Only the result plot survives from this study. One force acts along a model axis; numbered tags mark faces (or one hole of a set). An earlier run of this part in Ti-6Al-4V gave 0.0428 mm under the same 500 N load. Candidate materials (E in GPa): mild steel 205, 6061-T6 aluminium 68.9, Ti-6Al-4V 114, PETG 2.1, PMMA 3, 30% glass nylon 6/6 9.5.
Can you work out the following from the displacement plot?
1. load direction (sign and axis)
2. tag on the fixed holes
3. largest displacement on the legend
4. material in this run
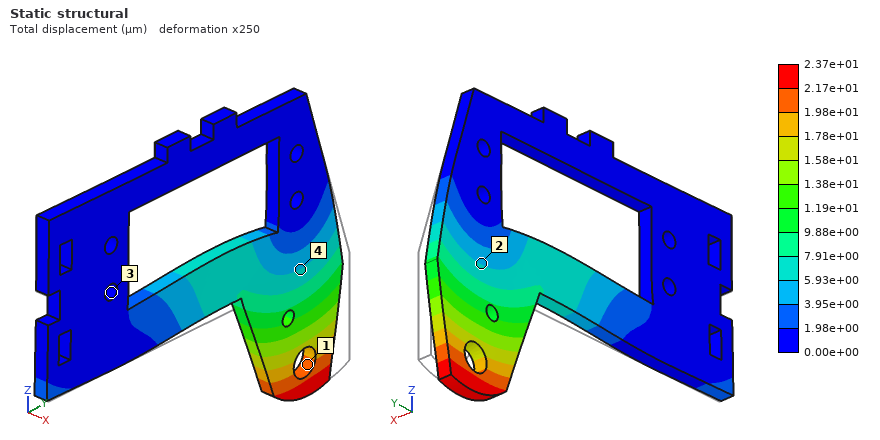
-Y
3
2.37e+01 µm
mild steel
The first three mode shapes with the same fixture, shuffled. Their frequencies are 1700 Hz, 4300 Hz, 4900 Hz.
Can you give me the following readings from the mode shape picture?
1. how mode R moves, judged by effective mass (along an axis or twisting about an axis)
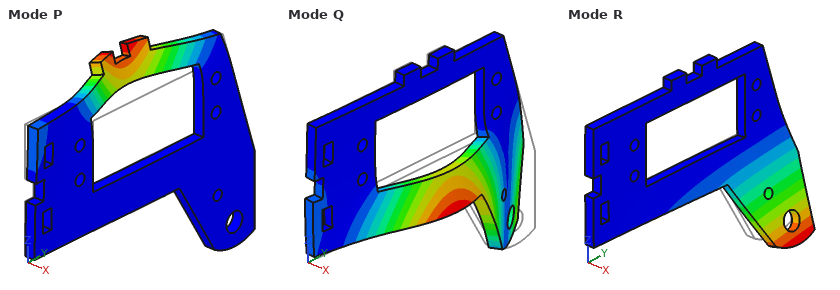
along X
